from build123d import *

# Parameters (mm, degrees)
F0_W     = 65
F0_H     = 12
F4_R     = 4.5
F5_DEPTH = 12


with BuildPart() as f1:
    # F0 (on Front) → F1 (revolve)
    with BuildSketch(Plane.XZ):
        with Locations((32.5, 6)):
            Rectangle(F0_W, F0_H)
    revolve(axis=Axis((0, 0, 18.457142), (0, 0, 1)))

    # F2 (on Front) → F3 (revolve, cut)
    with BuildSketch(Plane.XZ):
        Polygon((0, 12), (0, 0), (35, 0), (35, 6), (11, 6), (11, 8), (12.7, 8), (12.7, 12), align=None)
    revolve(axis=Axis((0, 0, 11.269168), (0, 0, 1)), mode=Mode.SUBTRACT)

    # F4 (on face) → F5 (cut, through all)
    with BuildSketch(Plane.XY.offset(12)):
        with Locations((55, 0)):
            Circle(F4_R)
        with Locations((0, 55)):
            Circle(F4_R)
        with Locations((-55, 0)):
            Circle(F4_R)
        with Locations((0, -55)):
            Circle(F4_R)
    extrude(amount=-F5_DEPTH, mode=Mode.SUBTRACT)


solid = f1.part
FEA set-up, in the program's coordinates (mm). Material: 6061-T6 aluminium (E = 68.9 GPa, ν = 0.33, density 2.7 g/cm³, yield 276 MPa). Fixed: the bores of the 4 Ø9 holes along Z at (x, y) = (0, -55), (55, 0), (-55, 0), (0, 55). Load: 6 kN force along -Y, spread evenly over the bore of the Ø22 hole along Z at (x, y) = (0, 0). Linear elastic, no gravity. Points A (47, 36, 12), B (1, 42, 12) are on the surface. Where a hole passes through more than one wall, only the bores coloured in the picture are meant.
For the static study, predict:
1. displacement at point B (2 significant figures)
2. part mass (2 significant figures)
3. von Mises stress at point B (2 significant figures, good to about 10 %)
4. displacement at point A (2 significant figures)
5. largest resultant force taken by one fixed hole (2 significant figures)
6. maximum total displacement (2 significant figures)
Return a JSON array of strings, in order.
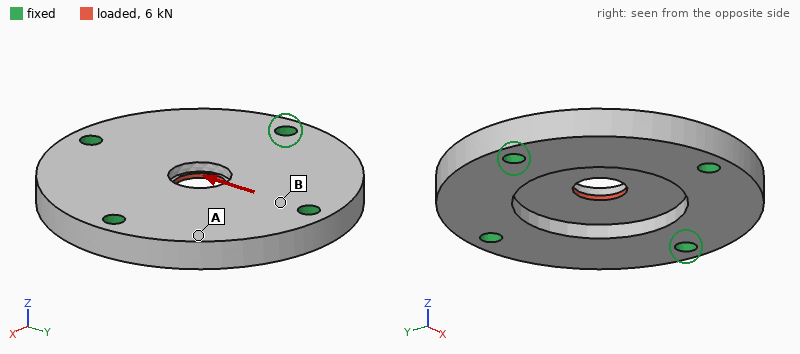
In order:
["2.5 µm", "350 g", "14 MPa", "2.5 µm", "1.9 kN", "11 µm"]
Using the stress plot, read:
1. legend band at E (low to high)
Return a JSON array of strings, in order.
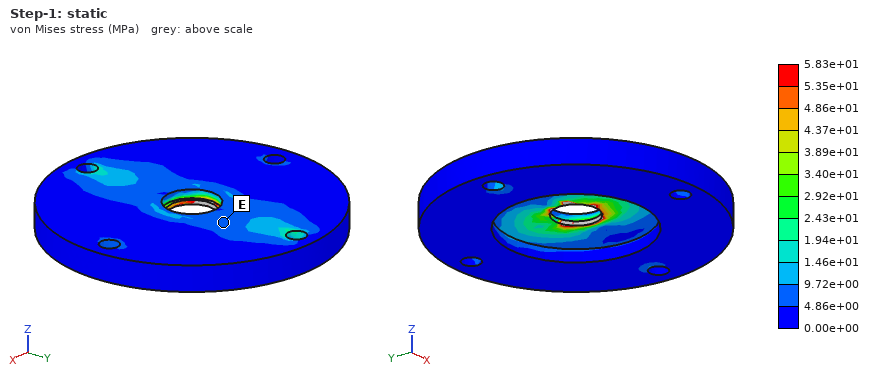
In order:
["4.86e+00 to 9.72e+00 MPa"]
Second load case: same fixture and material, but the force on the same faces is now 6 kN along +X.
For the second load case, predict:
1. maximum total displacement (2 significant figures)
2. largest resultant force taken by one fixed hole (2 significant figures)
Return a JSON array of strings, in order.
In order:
["11 µm", "1.9 kN"]
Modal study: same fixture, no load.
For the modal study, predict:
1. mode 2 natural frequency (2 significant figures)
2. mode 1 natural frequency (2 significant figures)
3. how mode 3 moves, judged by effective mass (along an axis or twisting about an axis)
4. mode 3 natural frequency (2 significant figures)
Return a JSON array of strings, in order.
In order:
["7400 Hz", "7300 Hz", "twisting about X", "7900 Hz"]
